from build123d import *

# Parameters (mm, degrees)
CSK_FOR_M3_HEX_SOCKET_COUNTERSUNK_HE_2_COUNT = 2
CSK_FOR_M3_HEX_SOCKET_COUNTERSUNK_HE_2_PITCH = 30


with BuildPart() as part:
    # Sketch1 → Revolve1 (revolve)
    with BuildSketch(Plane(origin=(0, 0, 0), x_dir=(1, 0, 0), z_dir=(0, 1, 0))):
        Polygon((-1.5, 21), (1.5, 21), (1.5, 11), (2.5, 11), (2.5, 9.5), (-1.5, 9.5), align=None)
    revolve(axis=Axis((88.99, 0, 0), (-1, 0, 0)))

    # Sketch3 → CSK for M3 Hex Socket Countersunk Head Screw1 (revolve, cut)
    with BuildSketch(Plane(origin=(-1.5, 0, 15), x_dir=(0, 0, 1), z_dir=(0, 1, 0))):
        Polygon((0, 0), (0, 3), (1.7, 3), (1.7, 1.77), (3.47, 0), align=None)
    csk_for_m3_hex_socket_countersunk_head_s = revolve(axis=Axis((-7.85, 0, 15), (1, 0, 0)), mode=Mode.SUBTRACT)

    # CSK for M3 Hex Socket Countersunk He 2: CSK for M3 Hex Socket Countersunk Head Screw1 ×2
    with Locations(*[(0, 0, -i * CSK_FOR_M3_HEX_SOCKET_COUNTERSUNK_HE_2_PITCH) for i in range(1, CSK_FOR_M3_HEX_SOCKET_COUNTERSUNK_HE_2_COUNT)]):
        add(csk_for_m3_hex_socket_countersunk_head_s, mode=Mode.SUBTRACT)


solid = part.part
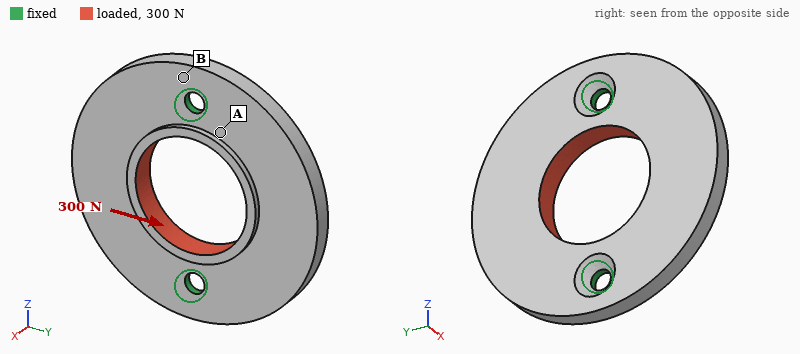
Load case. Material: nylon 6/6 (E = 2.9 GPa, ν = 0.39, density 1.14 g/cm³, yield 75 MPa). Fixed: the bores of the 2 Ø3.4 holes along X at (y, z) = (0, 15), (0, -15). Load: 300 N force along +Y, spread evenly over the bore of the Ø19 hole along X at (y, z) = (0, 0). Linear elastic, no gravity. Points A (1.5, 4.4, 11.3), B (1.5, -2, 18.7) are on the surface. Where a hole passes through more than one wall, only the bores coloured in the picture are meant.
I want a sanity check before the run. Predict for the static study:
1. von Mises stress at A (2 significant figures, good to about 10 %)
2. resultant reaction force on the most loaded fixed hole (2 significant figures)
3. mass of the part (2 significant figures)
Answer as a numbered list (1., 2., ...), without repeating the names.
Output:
1. 5.0 MPa
2. 150 N
3. 3.8 g
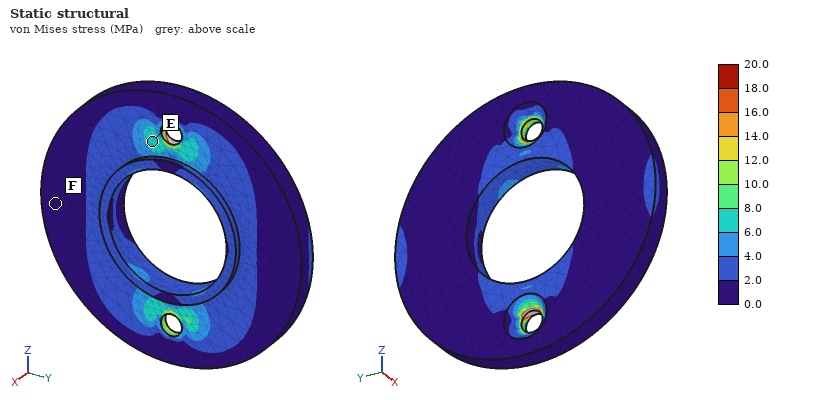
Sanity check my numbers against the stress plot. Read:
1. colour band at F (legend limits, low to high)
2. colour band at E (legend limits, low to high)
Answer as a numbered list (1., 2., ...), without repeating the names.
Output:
1. 0.0 to 2.0 MPa
2. 6.0 to 8.0 MPa
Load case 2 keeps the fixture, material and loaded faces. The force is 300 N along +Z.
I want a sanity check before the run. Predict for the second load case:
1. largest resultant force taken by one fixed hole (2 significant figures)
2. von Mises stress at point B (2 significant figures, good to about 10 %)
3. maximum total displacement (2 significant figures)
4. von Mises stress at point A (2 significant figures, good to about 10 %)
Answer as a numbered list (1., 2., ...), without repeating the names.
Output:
1. 150 N
2. 3.9 MPa
3. 33 µm
4. 6.3 MPa
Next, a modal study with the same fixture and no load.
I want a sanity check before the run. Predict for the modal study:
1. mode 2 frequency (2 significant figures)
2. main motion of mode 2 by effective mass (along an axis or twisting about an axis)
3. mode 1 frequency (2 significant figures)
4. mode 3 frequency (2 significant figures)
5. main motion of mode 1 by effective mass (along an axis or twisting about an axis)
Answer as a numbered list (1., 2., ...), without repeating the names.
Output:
1. 1600 Hz
2. along X
3. 1200 Hz
4. 3300 Hz
5. twisting about Z
